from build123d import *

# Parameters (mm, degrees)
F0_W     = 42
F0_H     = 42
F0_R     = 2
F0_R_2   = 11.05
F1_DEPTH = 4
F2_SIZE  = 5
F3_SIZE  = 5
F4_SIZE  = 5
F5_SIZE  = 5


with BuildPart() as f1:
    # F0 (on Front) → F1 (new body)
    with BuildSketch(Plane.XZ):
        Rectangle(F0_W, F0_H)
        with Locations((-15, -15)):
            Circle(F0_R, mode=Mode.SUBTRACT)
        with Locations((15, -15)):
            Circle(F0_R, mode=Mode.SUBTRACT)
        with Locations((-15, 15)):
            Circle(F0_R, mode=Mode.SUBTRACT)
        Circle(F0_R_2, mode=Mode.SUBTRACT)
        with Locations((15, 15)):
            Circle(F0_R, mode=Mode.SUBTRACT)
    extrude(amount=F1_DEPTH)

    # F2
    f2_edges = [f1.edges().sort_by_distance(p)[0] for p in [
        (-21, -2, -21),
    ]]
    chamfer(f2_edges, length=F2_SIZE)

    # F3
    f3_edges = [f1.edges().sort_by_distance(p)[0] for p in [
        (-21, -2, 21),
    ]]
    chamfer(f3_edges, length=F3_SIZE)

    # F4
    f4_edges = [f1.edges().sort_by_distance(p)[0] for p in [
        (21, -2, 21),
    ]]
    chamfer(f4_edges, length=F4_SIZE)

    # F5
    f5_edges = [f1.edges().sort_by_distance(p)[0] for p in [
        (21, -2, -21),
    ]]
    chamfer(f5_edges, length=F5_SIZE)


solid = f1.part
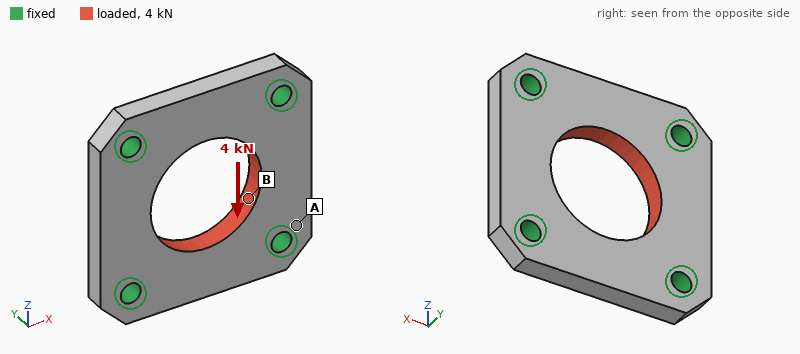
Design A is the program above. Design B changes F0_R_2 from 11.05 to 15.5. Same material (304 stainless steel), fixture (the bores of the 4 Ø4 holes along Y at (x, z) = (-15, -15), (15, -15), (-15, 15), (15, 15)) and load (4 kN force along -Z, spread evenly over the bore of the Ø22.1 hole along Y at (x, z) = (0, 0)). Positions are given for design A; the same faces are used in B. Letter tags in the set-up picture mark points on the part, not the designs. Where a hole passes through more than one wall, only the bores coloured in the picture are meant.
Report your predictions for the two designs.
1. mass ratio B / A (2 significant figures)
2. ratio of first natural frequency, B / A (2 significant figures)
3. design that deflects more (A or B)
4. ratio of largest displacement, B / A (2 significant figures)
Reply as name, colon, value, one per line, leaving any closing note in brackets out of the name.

mass ratio B / A: 0.71
ratio of first natural frequency, B / A: 1.0
design that deflects more: B
ratio of largest displacement, B / A: 1.5
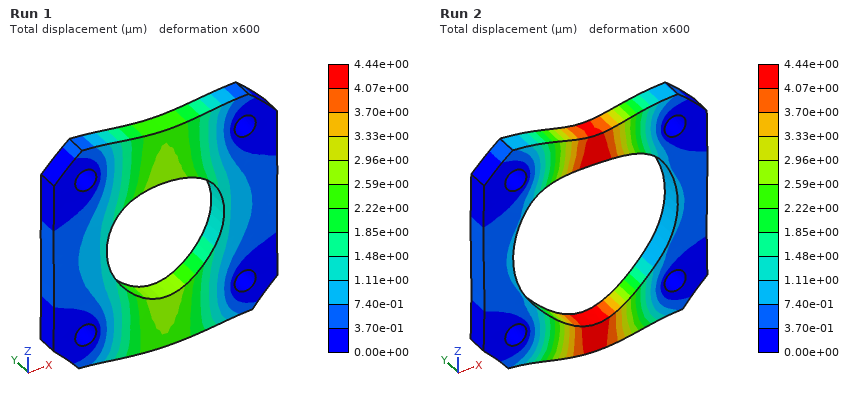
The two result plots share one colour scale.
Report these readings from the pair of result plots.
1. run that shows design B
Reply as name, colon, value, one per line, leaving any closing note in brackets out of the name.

run that shows design B: Run 2
